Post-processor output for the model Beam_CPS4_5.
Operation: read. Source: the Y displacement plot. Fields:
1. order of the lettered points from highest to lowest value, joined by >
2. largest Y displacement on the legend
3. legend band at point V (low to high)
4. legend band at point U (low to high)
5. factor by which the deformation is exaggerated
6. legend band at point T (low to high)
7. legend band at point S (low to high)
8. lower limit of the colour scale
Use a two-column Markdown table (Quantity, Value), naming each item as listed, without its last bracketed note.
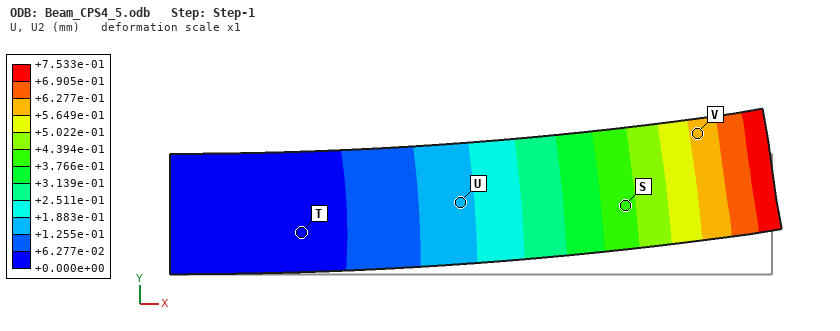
| Quantity | Value |
|---|---|
| order of the lettered points from highest to lowest value, joined by > | V > S > U > T |
| largest Y displacement on the legend | +7.533e-01 mm |
| legend band at point V | +5.649e-01 to +6.277e-01 mm |
| legend band at point U | +1.255e-01 to +1.883e-01 mm |
| factor by which the deformation is exaggerated | 1 |
| legend band at point T | +0.000e+00 to +6.277e-02 mm |
| legend band at point S | +3.766e-01 to +4.394e-01 mm |
| lower limit of the colour scale | +0.000e+00 mm |
